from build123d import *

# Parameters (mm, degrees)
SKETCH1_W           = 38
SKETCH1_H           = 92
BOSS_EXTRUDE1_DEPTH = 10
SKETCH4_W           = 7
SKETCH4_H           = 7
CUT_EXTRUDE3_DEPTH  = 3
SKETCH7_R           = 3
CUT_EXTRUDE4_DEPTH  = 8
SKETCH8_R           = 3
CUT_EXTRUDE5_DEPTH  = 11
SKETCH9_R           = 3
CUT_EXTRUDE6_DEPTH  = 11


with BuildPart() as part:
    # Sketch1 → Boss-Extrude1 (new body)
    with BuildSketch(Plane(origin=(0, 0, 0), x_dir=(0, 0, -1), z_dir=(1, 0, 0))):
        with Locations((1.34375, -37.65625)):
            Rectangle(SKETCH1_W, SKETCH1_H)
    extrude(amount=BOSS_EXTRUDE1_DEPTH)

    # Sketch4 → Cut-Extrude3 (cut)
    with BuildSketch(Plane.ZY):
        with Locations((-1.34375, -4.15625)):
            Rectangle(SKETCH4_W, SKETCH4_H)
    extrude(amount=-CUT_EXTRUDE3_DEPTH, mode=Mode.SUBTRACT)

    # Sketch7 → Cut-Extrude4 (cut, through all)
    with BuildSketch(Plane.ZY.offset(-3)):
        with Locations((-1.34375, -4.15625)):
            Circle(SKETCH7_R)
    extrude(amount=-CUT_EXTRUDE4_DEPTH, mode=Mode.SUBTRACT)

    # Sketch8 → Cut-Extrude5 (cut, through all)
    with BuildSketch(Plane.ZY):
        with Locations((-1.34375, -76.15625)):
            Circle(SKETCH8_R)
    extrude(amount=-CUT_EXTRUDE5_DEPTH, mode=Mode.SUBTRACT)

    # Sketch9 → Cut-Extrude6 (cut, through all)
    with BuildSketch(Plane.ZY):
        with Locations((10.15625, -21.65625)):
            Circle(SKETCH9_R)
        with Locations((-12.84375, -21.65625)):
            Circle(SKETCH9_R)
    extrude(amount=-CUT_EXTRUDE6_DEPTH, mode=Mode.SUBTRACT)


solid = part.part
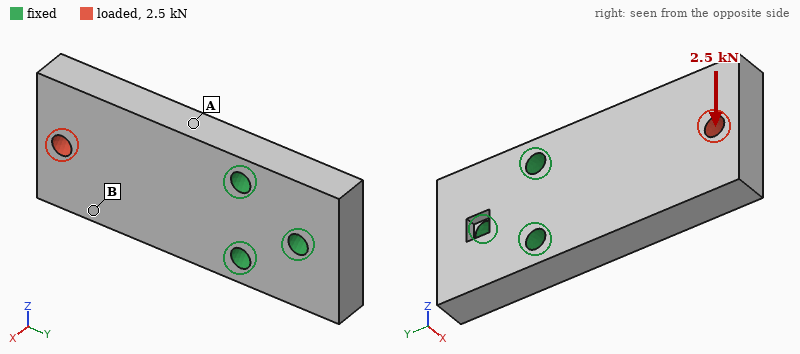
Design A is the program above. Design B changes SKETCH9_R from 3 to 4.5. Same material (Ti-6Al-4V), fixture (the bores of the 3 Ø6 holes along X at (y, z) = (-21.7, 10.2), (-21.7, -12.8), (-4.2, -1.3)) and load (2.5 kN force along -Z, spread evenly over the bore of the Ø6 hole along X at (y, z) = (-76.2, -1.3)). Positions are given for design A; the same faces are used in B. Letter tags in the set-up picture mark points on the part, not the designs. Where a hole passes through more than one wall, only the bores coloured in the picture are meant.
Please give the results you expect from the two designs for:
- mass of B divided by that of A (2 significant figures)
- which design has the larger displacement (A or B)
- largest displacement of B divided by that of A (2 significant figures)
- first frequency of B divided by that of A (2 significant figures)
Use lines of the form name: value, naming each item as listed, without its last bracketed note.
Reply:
mass of B divided by that of A: 0.98
which design has the larger displacement: A
largest displacement of B divided by that of A: 0.90
first frequency of B divided by that of A: 1.1
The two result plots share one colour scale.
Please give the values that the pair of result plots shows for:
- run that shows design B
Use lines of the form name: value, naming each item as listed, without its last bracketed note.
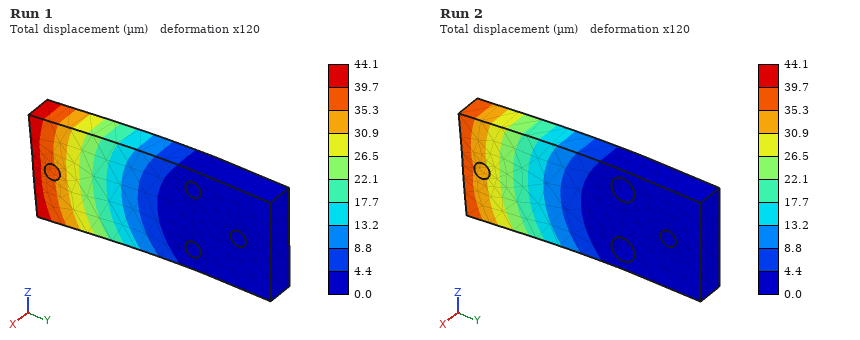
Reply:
run that shows design B: Run 2
